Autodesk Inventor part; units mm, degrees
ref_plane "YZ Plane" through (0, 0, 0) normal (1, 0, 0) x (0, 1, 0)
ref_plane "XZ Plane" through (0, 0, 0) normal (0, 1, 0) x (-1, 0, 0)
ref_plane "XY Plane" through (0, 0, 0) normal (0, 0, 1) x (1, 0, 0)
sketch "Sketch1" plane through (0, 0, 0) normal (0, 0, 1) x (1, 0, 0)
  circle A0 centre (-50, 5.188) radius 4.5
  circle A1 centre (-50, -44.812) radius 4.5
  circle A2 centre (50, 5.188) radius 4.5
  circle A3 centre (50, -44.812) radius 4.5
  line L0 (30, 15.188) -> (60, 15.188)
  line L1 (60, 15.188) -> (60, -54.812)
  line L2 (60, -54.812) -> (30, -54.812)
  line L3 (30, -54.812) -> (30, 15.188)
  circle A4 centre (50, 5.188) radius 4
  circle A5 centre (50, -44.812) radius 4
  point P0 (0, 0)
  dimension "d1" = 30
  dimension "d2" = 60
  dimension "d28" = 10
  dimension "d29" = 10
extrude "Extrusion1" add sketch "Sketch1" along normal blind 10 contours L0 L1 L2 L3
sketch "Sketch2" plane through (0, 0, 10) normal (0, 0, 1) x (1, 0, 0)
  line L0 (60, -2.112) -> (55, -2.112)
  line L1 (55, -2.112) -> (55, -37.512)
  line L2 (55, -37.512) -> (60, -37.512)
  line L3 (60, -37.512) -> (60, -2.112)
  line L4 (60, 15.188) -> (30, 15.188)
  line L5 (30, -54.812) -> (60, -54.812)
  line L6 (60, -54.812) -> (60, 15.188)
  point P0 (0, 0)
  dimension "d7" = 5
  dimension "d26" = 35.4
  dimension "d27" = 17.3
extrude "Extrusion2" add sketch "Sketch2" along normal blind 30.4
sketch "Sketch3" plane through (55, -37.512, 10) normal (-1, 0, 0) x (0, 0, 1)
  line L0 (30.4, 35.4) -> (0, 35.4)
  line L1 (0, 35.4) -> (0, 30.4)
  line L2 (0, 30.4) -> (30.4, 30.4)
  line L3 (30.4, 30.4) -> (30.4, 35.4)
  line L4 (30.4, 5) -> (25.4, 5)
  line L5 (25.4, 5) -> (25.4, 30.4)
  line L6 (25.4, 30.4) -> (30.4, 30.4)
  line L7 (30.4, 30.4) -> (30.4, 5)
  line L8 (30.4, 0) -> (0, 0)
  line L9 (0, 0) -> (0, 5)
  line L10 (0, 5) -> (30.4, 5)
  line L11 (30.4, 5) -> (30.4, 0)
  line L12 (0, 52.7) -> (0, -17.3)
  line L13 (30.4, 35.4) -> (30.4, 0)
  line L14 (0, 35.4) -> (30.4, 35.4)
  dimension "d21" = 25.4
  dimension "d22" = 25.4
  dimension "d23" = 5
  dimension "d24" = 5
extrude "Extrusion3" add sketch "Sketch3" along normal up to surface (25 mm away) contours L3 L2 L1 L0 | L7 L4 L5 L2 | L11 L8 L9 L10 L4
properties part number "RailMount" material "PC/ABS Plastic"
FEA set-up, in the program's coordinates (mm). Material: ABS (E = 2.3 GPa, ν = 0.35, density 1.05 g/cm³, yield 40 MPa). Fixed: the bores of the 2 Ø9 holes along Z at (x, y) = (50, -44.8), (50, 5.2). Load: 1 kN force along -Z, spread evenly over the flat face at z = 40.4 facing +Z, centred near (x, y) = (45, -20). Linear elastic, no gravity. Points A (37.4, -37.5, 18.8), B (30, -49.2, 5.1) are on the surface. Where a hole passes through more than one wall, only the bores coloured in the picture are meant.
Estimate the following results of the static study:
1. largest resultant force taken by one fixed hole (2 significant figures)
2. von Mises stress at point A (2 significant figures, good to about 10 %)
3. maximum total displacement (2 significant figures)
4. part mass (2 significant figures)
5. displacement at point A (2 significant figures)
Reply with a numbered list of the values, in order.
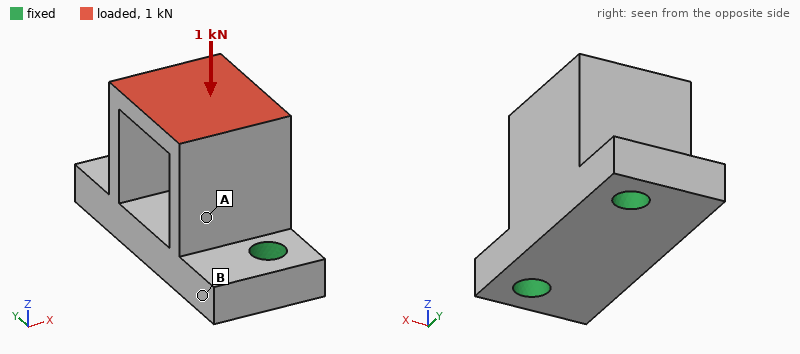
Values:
1. 510 N
2. 4.4 MPa
3. 0.33 mm
4. 38 g
5. 0.091 mm
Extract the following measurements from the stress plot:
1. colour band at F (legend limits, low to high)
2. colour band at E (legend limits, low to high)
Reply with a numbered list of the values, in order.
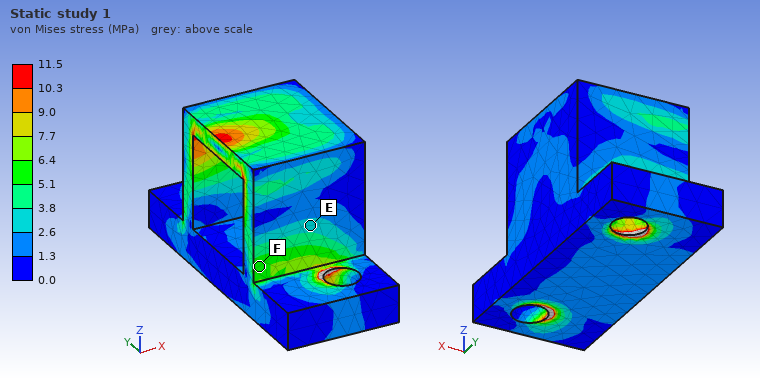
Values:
1. 5.1 to 6.4 MPa
2. 2.6 to 3.8 MPa
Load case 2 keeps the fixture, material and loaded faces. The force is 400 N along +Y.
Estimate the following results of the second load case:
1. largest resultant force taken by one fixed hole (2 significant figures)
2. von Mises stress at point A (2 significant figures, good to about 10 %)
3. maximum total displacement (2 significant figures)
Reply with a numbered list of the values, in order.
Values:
1. 400 N
2. 5.1 MPa
3. 0.43 mm
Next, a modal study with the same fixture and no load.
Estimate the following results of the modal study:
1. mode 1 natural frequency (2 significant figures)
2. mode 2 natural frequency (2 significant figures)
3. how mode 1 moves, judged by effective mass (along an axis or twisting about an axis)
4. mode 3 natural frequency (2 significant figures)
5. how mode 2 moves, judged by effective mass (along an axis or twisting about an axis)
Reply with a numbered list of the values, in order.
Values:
1. 1600 Hz
2. 1900 Hz
3. along X
4. 4100 Hz
5. along Y
